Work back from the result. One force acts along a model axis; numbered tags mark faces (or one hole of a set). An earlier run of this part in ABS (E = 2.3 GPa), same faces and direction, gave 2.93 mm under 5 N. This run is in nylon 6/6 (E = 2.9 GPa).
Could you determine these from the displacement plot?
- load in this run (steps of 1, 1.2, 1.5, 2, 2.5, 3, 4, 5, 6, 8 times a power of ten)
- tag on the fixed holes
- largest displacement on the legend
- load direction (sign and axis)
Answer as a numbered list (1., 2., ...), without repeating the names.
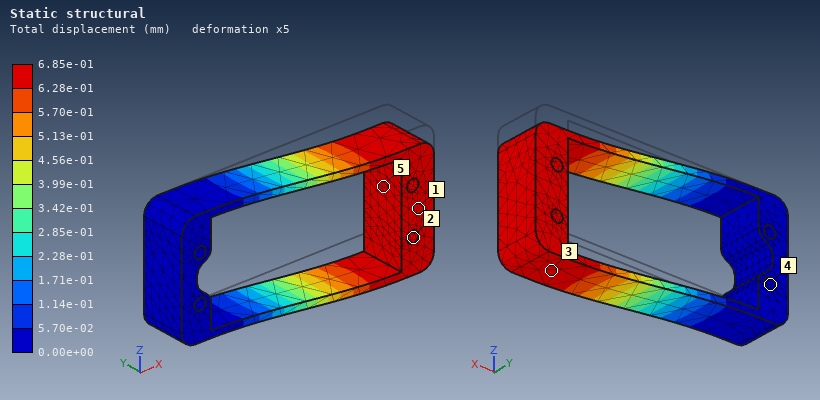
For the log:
1. 1.5 N
2. 4
3. 6.85e-01 mm
4. -Z
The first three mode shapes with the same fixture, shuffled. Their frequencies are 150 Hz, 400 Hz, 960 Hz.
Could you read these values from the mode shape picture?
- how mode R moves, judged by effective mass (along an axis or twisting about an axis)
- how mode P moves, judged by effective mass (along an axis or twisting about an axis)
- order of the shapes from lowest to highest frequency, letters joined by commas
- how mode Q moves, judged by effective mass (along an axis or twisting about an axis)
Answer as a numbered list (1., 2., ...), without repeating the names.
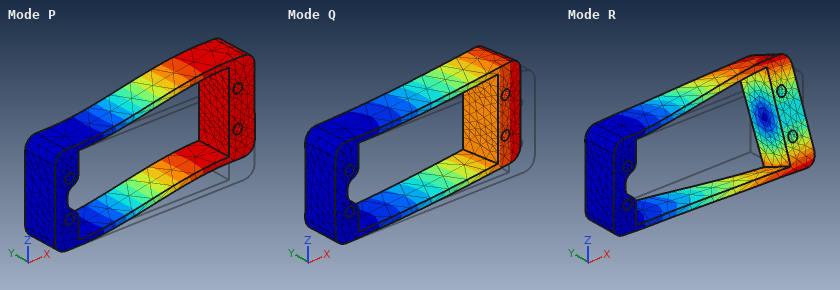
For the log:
1. twisting about X
2. along Z
3. P, Q, R
4. along Y
